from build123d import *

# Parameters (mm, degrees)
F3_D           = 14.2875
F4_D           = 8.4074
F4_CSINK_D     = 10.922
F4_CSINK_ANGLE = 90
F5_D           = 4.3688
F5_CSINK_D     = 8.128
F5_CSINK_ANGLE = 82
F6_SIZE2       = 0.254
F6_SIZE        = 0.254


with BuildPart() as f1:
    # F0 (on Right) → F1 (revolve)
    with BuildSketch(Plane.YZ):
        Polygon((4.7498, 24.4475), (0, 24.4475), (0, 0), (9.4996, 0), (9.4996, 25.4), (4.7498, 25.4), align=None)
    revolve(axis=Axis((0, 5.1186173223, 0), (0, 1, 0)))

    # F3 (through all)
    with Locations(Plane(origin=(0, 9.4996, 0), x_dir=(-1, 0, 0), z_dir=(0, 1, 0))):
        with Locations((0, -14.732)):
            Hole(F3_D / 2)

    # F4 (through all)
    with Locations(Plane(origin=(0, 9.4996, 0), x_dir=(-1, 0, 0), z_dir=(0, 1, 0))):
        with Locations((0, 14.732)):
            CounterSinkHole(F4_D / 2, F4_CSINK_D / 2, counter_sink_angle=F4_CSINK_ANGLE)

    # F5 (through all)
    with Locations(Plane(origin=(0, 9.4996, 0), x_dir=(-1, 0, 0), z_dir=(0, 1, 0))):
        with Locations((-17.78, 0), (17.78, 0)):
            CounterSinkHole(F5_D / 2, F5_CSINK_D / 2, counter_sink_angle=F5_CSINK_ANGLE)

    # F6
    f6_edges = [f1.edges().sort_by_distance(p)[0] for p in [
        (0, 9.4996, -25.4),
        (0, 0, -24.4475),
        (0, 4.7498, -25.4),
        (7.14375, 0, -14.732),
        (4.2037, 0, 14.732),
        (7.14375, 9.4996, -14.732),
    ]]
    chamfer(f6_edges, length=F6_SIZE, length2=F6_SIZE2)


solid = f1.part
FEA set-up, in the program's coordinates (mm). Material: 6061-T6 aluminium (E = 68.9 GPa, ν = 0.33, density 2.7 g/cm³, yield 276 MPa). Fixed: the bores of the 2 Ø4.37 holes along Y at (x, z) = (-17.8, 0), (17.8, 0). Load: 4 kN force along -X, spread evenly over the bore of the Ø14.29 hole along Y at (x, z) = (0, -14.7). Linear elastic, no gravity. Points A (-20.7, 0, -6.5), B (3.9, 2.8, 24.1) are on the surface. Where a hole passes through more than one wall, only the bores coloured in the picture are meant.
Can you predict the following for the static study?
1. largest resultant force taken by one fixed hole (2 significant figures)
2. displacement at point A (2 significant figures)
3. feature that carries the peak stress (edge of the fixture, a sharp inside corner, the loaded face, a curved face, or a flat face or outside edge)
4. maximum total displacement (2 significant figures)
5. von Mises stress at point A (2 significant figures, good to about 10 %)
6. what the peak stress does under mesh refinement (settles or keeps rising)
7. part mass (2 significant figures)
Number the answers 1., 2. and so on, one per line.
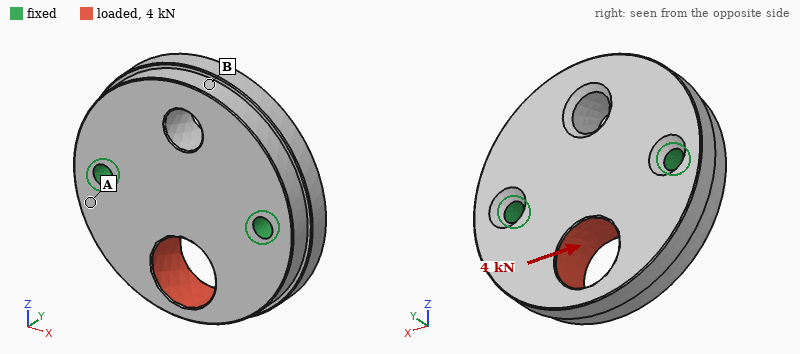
1. 2.5 kN
2. 3.9 µm
3. edge of the fixture
4. 18 µm
5. 16 MPa
6. keeps rising
7. 43 g
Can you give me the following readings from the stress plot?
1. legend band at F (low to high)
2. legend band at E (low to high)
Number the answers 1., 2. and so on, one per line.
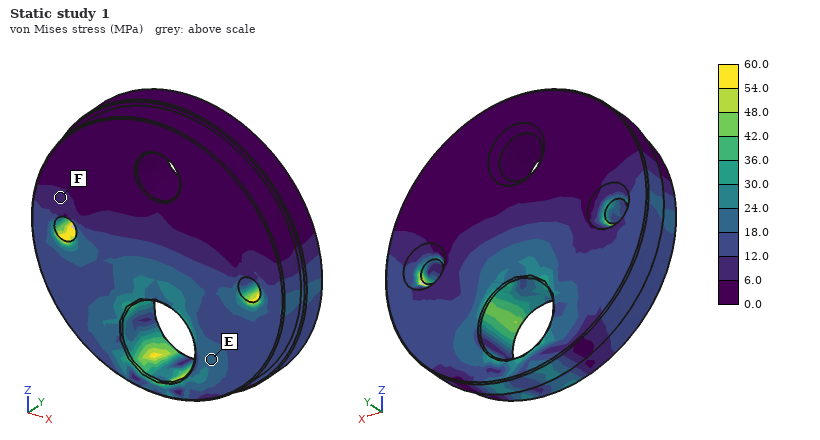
1. 6.0 to 12.0 MPa
2. 18.0 to 24.0 MPa
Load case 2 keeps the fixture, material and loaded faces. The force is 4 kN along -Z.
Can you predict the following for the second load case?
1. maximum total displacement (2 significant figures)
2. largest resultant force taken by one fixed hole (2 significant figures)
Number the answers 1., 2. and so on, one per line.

1. 12 µm
2. 2.1 kN
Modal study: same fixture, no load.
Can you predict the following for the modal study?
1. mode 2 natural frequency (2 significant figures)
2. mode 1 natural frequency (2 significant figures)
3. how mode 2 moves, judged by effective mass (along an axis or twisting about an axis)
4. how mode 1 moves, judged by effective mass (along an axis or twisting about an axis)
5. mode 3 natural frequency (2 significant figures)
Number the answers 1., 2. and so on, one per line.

1. 13 kHz
2. 9400 Hz
3. along Y
4. twisting about X
5. 21 kHz
